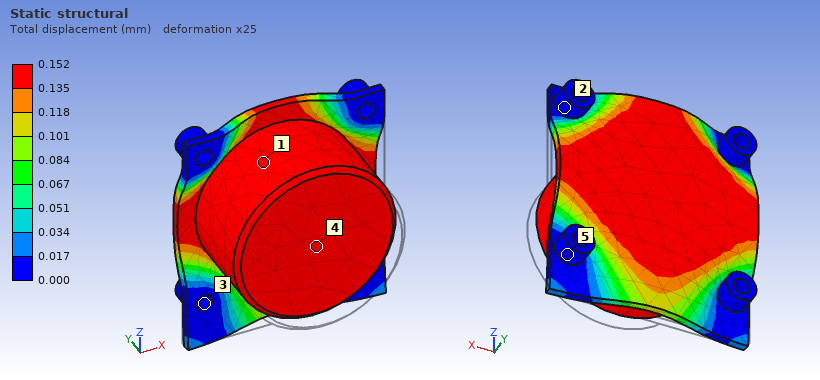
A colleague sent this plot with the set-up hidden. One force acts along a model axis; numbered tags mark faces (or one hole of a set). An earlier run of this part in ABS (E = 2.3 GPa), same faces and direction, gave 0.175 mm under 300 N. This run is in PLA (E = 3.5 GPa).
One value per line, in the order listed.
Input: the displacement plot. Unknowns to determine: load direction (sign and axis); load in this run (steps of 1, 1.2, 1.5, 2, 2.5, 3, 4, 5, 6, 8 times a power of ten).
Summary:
+Y
400 N
